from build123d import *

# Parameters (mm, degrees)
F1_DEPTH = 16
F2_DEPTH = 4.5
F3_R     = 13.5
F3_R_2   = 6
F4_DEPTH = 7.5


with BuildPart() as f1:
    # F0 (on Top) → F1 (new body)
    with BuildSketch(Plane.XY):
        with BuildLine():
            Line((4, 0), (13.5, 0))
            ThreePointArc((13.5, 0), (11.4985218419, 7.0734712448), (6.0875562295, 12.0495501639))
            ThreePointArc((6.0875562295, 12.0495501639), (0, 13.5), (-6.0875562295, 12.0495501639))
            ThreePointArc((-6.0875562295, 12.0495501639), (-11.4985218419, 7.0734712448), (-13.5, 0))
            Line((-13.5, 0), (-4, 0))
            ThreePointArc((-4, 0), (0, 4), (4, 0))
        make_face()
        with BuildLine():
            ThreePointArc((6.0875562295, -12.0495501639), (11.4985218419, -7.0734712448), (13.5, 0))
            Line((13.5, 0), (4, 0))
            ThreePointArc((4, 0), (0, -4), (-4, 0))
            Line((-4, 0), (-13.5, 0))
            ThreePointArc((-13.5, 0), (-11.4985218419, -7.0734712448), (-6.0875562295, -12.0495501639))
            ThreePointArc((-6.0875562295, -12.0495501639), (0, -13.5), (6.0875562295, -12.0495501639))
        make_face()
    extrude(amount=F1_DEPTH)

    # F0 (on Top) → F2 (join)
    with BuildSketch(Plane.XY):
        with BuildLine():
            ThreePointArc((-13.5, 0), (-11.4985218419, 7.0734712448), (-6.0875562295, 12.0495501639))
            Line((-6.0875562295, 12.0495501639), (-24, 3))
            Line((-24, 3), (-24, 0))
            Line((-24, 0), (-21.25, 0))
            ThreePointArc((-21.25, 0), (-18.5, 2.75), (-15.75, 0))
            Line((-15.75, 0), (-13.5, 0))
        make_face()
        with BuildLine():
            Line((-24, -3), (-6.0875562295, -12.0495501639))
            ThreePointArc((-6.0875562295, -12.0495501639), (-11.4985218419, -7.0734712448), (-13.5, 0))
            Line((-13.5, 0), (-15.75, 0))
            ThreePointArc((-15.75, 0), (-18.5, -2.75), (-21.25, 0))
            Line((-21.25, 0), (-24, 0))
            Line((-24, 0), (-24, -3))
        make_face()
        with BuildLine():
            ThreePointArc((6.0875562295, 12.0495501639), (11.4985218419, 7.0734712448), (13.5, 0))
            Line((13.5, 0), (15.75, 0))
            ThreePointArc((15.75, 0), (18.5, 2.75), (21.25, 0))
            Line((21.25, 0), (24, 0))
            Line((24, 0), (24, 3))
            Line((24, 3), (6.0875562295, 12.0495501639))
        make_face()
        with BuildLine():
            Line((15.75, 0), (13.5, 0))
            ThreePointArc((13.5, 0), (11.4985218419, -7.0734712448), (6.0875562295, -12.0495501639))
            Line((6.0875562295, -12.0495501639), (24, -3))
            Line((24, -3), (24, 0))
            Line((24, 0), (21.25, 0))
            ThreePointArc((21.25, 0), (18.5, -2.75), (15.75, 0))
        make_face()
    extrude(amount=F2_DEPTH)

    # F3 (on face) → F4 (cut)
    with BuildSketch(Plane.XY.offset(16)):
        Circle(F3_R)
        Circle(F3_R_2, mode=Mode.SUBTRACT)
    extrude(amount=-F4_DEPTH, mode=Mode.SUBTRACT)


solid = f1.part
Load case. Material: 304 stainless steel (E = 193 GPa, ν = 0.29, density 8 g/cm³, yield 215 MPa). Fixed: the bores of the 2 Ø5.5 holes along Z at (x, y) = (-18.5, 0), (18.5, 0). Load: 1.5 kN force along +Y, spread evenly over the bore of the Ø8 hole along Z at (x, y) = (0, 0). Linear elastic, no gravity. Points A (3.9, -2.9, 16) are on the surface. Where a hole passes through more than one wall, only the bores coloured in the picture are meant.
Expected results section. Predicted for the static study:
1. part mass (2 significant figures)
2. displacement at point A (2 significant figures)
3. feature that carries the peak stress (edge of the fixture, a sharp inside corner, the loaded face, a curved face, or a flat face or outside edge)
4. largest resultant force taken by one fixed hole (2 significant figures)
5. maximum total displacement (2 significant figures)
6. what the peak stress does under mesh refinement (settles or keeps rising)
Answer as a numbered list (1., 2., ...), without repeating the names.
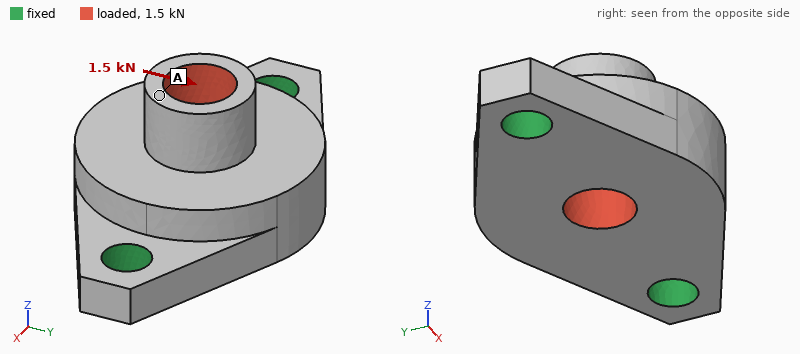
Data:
1. 48 g
2. 14 µm
3. edge of the fixture
4. 750 N
5. 15 µm
6. keeps rising
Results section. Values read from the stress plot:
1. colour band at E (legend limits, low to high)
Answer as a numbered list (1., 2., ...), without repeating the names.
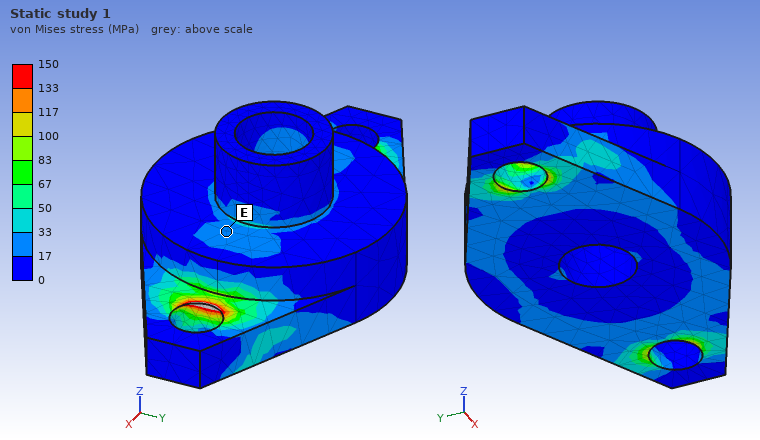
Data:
1. 17 to 33 MPa
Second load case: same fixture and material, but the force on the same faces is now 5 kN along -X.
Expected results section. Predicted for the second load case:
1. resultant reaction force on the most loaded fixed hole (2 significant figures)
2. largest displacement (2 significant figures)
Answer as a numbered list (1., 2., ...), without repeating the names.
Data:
1. 2.7 kN
2. 11 µm
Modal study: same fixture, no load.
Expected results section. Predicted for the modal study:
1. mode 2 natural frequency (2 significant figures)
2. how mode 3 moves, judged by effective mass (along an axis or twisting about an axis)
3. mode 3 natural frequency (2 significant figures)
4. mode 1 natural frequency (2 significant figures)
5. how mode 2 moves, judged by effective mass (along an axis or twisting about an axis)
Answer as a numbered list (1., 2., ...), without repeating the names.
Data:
1. 16 kHz
2. along Y
3. 27 kHz
4. 11 kHz
5. along Z
